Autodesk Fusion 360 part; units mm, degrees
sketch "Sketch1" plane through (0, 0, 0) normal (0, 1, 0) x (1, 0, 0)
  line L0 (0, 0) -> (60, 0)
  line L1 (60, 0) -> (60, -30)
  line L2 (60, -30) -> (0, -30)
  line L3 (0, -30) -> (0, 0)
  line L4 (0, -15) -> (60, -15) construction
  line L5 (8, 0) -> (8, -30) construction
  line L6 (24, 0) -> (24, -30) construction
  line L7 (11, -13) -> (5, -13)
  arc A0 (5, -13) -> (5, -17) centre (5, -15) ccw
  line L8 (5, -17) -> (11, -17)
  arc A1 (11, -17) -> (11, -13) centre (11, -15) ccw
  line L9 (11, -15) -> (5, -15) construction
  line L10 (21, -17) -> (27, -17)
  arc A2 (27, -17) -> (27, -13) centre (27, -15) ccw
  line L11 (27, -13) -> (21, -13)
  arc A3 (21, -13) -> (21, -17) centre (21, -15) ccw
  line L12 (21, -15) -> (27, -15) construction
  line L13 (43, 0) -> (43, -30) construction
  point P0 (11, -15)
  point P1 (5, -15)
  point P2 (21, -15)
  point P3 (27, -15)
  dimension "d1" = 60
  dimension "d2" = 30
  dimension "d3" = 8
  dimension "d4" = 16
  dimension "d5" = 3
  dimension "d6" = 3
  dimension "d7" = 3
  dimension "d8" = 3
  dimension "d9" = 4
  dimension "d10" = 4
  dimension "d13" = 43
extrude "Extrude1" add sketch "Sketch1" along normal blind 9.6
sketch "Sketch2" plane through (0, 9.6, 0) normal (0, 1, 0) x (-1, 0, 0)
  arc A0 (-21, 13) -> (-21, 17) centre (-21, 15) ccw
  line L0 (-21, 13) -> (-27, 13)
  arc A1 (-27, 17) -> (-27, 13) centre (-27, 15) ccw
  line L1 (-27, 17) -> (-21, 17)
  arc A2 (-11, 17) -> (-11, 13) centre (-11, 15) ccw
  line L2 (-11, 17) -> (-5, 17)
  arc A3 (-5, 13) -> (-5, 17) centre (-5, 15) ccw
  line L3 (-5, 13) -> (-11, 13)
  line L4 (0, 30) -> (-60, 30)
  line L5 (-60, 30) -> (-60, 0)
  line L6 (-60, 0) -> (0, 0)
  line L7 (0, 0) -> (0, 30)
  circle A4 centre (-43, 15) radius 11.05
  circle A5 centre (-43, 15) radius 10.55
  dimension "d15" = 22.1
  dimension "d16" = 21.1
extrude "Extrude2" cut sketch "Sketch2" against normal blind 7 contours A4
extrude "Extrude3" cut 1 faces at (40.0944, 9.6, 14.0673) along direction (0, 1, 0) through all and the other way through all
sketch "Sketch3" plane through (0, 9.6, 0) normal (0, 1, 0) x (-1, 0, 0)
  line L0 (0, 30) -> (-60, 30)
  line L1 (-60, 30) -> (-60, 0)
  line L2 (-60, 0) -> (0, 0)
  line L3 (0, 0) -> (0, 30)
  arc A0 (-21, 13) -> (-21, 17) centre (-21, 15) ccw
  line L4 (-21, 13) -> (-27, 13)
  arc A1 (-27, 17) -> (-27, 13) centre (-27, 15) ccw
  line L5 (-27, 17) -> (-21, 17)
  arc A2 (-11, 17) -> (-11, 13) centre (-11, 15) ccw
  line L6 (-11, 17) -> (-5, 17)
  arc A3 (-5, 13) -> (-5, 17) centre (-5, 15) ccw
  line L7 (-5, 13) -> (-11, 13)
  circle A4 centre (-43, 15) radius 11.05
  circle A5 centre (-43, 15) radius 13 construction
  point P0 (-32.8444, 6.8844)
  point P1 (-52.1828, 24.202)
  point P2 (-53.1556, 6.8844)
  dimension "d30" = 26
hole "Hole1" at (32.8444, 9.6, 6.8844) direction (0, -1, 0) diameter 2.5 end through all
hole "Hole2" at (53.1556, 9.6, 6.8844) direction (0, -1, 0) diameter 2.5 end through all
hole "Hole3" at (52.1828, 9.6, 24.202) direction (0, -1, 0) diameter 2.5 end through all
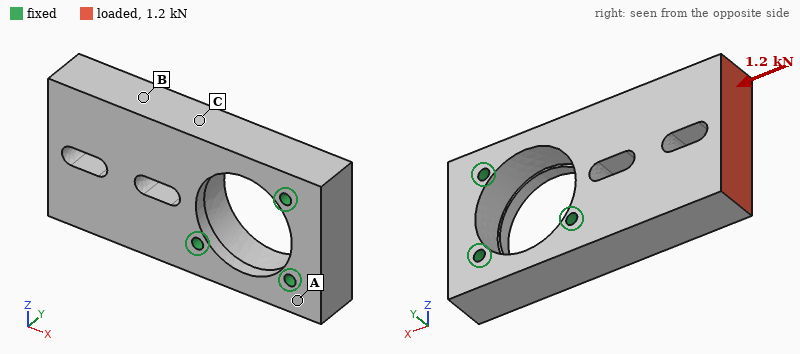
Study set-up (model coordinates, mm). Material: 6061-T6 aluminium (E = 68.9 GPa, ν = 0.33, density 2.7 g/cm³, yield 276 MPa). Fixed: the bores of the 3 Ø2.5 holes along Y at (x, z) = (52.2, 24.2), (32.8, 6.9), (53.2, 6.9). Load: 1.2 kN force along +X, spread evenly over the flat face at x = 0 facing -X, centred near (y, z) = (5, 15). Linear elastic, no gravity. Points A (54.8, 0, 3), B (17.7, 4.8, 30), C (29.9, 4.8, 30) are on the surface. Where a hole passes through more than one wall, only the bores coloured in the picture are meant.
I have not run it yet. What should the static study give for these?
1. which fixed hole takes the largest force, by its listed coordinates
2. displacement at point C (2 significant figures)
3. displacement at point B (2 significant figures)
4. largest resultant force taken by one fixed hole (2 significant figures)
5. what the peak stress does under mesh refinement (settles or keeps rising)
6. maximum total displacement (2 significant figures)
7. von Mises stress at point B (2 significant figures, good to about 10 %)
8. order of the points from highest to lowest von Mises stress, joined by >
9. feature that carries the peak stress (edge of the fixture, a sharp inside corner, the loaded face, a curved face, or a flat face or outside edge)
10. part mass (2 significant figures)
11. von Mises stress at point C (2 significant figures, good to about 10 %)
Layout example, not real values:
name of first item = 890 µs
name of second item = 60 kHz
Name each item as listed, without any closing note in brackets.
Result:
which fixed hole takes the largest force, by its listed coordinates = (32.8, 6.9)
displacement at point C = 4.1 µm
displacement at point B = 6.0 µm
largest resultant force taken by one fixed hole = 730 N
what the peak stress does under mesh refinement = keeps rising
maximum total displacement = 8.5 µm
von Mises stress at point B = 6.2 MPa
order of the points from highest to lowest von Mises stress, joined by > = C > B > A
feature that carries the peak stress = edge of the fixture
part mass = 35 g
von Mises stress at point C = 11 MPa
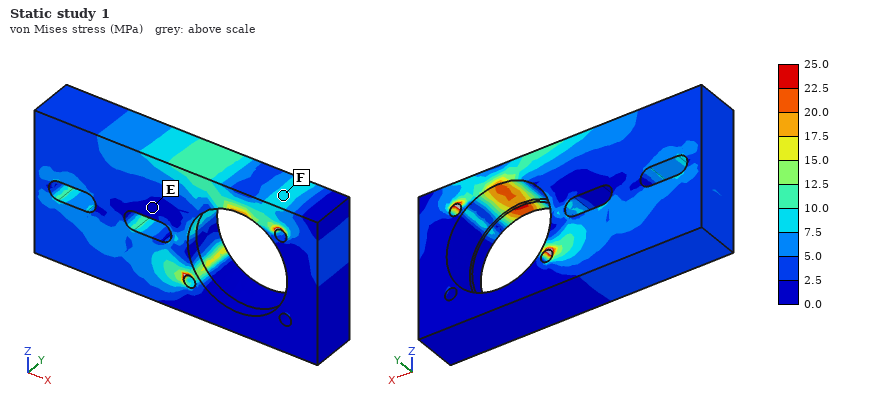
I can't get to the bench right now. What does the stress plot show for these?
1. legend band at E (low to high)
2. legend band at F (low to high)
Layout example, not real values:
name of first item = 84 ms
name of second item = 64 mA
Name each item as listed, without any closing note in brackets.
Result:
legend band at E = 0.0 to 2.5 MPa
legend band at F = 7.5 to 10.0 MPa
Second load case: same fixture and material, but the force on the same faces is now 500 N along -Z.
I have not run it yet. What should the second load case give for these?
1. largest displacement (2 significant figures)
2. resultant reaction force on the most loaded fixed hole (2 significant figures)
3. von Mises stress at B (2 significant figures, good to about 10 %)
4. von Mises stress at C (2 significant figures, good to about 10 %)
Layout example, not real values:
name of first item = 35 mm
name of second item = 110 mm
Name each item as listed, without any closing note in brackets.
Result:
largest displacement = 21 µm
resultant reaction force on the most loaded fixed hole = 740 N
von Mises stress at B = 8.0 MPa
von Mises stress at C = 17 MPa
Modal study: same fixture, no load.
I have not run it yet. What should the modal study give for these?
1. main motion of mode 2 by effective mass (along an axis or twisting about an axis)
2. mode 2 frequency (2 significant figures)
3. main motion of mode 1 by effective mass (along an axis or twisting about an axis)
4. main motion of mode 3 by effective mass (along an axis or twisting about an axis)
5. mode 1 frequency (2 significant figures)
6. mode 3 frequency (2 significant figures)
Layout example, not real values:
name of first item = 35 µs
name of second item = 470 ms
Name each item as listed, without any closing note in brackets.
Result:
main motion of mode 2 by effective mass = along Z
mode 2 frequency = 8700 Hz
main motion of mode 1 by effective mass = along Y
main motion of mode 3 by effective mass = twisting about X
mode 1 frequency = 4300 Hz
mode 3 frequency = 9700 Hz
